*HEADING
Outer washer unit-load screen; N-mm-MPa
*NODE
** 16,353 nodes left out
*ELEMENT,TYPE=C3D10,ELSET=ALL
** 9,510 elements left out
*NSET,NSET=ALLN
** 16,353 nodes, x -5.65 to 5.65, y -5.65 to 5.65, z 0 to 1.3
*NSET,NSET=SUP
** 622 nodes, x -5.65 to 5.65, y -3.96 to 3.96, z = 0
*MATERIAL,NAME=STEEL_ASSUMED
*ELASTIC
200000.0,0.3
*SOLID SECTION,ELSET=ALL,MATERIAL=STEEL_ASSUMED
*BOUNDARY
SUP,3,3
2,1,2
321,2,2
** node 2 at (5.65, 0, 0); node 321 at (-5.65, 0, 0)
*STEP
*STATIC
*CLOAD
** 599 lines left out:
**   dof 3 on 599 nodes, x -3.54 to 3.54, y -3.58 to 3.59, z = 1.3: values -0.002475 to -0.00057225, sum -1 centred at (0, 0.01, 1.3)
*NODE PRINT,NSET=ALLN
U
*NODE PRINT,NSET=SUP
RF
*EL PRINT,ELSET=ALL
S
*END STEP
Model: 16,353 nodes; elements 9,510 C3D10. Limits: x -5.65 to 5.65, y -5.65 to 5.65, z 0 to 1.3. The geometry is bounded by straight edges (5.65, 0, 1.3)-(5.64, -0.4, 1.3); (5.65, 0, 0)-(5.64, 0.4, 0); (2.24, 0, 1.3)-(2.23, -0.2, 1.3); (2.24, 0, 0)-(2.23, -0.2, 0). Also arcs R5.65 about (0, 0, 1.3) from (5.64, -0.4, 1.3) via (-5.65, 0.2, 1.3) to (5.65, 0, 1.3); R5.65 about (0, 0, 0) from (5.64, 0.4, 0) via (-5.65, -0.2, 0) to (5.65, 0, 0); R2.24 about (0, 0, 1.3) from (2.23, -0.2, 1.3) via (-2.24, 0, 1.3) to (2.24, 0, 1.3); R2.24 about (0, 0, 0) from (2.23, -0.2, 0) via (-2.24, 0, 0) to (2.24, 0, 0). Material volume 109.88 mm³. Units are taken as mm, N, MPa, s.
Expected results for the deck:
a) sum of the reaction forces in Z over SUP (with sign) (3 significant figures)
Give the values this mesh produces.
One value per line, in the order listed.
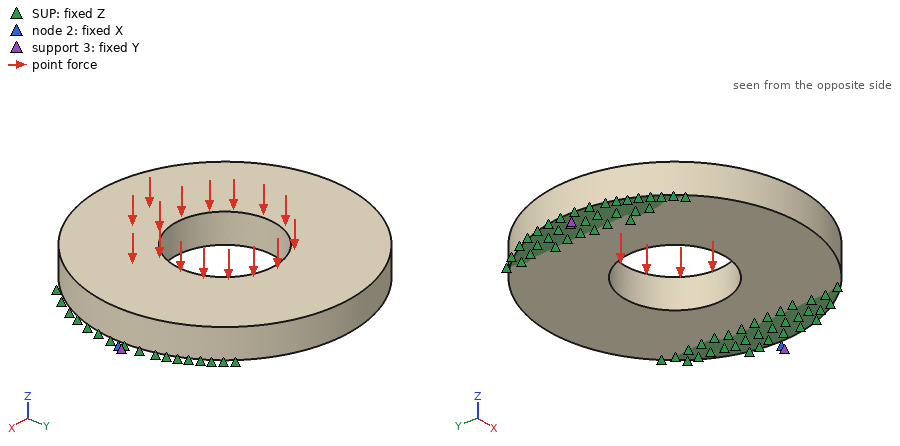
1.00 N
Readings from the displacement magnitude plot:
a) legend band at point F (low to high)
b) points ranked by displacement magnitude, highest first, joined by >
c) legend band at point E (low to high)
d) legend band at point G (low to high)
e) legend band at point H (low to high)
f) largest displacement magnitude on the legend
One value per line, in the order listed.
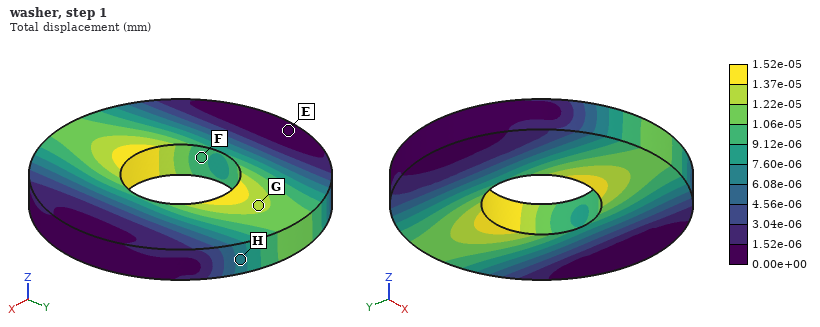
9.12e-06 to 1.06e-05 mm
G > F > H > E
0.00e+00 to 1.52e-06 mm
1.22e-05 to 1.37e-05 mm
6.08e-06 to 7.60e-06 mm
1.52e-05 mm
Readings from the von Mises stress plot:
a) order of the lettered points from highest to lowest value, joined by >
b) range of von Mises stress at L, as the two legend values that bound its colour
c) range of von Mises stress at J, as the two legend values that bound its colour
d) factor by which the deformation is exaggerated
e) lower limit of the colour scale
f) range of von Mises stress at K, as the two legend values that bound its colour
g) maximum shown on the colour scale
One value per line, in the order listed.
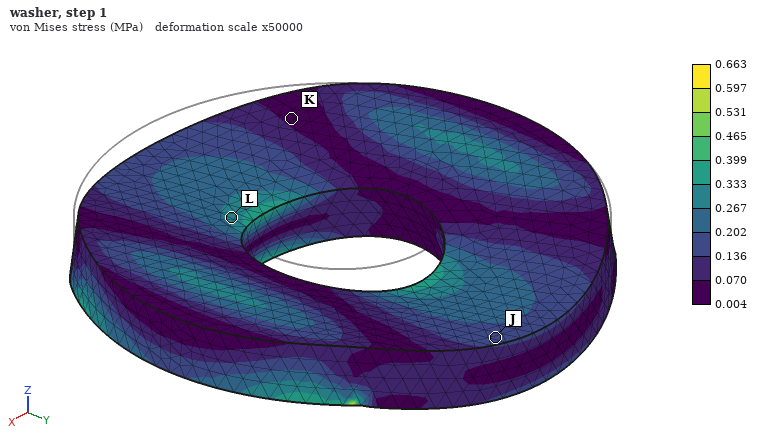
L > J > K
0.267 to 0.333 MPa
0.136 to 0.202 MPa
50000
0.004 MPa
0.004 to 0.070 MPa
0.663 MPa
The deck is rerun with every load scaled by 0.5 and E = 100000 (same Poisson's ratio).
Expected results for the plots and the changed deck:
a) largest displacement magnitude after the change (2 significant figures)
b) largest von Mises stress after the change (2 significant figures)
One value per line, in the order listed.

1.5e-05 mm
0.33 MPa
